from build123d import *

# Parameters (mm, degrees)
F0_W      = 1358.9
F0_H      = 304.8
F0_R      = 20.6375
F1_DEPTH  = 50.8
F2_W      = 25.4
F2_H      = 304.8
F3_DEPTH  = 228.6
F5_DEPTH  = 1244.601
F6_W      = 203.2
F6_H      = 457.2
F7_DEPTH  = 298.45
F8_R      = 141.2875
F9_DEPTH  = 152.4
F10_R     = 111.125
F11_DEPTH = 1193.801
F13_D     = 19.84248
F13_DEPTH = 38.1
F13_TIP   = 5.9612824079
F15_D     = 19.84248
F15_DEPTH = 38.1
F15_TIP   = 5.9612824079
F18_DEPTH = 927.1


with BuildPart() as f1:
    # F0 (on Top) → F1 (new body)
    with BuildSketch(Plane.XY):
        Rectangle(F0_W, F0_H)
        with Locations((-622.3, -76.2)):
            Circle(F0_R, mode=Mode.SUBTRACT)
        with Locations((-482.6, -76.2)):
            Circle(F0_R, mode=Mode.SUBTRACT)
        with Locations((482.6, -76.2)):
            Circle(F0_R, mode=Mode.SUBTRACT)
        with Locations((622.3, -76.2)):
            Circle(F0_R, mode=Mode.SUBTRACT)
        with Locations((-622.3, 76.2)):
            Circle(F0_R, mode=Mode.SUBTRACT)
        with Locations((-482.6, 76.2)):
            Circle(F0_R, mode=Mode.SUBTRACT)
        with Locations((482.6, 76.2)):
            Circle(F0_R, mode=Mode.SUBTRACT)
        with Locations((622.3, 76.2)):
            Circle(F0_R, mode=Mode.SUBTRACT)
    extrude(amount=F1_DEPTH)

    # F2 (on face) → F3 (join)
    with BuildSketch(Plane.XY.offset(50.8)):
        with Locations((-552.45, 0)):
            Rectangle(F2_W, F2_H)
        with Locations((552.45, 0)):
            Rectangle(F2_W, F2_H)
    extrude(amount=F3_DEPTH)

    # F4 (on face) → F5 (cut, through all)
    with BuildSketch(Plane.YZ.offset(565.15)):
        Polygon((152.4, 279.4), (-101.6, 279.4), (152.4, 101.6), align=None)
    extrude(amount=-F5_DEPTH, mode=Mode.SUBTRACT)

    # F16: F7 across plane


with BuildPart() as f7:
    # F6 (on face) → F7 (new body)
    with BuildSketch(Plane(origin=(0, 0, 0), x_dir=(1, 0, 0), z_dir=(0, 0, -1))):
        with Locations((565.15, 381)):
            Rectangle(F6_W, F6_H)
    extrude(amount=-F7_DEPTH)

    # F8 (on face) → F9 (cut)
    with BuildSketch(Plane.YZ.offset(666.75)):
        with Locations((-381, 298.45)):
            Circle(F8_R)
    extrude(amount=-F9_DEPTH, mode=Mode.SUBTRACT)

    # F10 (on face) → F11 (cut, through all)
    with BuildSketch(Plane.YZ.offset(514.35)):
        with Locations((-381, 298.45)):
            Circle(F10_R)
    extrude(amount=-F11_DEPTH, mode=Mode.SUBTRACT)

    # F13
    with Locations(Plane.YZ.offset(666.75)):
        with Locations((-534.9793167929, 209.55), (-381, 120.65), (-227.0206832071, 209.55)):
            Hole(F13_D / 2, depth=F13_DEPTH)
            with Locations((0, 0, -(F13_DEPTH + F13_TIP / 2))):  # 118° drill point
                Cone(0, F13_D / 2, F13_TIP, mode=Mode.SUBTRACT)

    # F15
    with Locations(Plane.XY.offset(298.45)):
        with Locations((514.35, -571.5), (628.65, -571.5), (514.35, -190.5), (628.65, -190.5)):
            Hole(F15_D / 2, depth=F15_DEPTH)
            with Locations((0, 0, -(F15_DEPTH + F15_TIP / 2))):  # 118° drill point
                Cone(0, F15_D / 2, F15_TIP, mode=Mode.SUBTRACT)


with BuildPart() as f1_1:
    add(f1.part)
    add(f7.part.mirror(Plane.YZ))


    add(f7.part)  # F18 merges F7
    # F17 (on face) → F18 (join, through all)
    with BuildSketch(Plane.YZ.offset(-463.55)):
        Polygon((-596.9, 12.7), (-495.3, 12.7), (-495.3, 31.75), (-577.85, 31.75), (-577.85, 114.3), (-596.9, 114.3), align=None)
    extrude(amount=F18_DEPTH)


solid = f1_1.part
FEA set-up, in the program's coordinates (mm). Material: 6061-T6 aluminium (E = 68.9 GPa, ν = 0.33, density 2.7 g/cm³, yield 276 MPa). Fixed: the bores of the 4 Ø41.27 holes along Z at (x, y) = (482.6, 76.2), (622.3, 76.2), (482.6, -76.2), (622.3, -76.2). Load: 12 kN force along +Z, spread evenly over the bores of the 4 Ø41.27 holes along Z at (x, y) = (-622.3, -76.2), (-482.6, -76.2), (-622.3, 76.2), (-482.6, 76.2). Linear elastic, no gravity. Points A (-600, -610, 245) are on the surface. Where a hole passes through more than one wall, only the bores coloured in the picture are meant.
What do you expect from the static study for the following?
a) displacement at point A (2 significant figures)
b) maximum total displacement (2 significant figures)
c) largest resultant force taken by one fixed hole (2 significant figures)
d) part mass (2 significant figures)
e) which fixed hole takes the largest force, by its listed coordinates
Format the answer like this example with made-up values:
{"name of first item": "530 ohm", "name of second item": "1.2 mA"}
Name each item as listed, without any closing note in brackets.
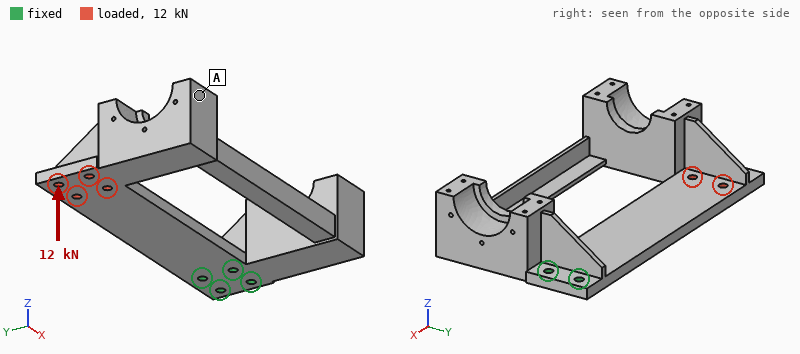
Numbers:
{"displacement at point A": "9.9 mm", "maximum total displacement": "14 mm", "largest resultant force taken by one fixed hole": "39 kN", "part mass": "190 kg", "which fixed hole takes the largest force, by its listed coordinates": "(482.6, -76.2)"}
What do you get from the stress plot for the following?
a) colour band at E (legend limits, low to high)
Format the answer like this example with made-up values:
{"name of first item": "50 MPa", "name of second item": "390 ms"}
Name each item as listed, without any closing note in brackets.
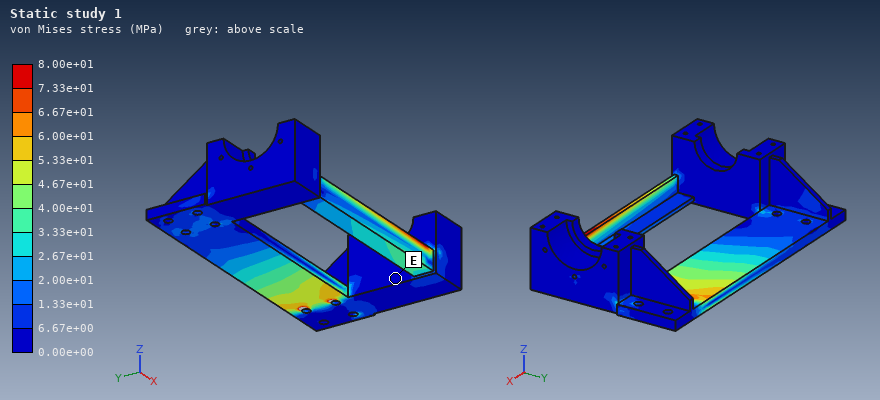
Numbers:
{"colour band at E": "0.00e+00 to 6.67e+00 MPa"}
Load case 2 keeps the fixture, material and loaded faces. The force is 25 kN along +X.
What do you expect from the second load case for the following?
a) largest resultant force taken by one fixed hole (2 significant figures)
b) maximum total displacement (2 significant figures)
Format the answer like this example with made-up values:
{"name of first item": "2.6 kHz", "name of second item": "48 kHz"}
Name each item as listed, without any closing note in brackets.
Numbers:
{"largest resultant force taken by one fixed hole": "12 kN", "maximum total displacement": "30 µm"}
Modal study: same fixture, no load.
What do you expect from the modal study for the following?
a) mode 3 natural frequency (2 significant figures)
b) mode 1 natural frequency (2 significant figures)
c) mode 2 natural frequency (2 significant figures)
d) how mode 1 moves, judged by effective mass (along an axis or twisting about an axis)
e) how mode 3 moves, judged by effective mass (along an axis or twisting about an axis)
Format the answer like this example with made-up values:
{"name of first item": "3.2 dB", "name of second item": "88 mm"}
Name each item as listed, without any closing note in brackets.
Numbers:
{"mode 3 natural frequency": "100 Hz", "mode 1 natural frequency": "19 Hz", "mode 2 natural frequency": "56 Hz", "how mode 1 moves, judged by effective mass": "along Z", "how mode 3 moves, judged by effective mass": "along Y"}
